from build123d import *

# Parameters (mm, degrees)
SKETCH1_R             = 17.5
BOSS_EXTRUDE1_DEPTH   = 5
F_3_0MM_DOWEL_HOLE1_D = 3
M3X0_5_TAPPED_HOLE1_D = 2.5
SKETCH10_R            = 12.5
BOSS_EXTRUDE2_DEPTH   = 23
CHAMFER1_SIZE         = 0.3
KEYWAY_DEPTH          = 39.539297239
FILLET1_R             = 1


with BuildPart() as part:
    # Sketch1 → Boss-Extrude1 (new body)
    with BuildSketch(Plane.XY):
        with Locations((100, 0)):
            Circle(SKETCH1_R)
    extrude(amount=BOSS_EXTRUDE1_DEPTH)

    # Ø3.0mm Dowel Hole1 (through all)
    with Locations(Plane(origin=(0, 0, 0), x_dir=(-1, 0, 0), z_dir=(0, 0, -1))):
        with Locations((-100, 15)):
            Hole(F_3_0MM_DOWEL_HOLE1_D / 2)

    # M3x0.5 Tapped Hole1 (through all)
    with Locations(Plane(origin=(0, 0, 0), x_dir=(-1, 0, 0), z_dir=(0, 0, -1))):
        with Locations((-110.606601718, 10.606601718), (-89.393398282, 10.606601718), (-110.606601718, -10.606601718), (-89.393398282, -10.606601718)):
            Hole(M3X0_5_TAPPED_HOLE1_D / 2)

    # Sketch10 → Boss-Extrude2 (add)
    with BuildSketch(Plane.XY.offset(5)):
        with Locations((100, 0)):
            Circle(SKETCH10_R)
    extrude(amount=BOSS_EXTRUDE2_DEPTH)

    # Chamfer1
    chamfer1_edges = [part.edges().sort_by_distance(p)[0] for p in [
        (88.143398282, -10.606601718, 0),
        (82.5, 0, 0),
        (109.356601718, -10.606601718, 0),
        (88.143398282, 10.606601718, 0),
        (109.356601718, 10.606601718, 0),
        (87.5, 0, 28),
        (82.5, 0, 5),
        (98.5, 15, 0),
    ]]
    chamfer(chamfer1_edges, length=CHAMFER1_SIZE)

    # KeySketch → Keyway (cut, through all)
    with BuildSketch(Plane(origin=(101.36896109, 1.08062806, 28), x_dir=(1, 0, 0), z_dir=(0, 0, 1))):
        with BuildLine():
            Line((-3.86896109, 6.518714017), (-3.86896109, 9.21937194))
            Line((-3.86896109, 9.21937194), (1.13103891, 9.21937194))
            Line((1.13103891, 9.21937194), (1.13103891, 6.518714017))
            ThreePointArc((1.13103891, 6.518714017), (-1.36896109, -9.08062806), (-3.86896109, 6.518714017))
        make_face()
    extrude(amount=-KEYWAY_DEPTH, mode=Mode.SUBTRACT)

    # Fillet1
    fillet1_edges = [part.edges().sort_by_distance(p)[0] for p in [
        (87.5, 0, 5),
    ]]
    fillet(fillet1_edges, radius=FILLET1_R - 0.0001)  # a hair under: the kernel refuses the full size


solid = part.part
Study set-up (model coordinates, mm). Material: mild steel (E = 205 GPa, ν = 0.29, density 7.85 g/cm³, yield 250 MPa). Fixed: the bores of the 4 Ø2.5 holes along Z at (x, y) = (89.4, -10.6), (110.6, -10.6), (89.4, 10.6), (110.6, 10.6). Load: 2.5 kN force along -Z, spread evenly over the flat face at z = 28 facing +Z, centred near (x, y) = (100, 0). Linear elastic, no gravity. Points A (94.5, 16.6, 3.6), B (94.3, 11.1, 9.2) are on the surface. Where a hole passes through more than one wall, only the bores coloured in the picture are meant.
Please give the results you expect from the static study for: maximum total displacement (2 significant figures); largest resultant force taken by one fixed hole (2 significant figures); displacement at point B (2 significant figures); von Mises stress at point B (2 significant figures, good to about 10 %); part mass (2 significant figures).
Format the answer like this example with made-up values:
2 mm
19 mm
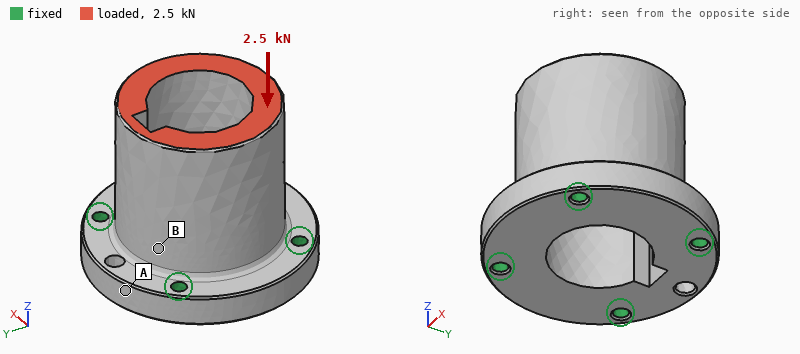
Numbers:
2.1 µm
680 N
1.3 µm
12 MPa
78 g
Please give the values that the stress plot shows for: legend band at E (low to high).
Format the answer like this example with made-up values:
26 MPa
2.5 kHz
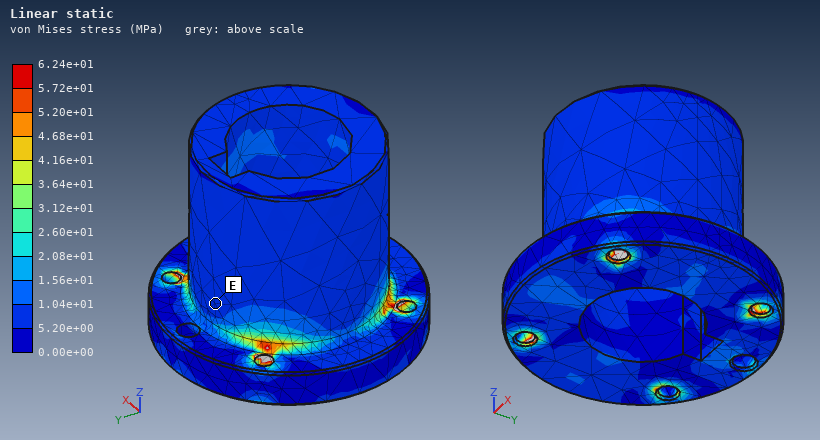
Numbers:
5.20e+00 to 1.04e+01 MPa
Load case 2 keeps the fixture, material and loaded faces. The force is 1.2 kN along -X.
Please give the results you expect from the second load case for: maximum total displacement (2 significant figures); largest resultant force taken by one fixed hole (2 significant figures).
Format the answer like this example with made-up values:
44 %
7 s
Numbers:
8.9 µm
840 N
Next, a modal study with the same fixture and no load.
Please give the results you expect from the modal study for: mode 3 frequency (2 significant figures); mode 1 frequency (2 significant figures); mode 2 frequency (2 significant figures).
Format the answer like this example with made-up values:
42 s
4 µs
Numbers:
24 kHz
14 kHz
15 kHz
